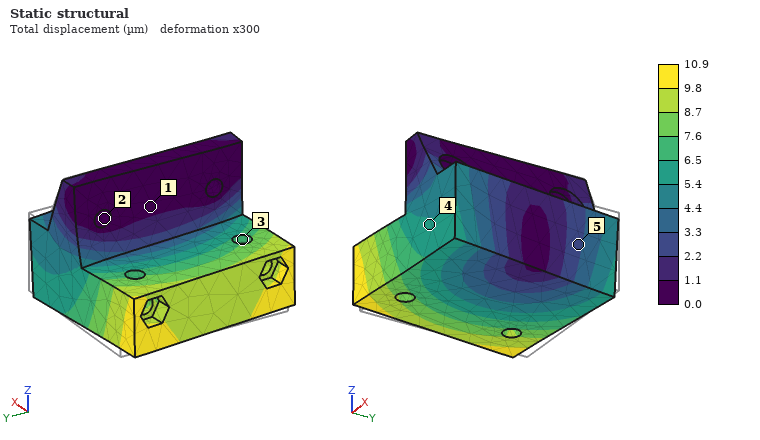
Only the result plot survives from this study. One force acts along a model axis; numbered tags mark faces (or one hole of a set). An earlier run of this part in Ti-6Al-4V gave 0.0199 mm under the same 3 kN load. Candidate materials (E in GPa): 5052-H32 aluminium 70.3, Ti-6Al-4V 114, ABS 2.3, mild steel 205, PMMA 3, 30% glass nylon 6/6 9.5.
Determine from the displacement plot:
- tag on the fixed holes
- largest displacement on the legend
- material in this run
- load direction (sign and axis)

2
10.9 µm
mild steel
-Y
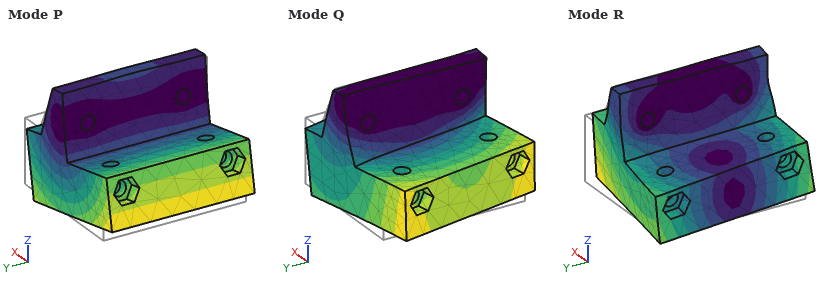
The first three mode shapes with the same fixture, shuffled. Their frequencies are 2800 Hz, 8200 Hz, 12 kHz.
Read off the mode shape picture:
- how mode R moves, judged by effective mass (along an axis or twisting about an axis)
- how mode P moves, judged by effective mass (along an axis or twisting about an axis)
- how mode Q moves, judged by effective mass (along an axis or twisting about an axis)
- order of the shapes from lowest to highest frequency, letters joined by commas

along Y
along X
along Y
P, Q, R
